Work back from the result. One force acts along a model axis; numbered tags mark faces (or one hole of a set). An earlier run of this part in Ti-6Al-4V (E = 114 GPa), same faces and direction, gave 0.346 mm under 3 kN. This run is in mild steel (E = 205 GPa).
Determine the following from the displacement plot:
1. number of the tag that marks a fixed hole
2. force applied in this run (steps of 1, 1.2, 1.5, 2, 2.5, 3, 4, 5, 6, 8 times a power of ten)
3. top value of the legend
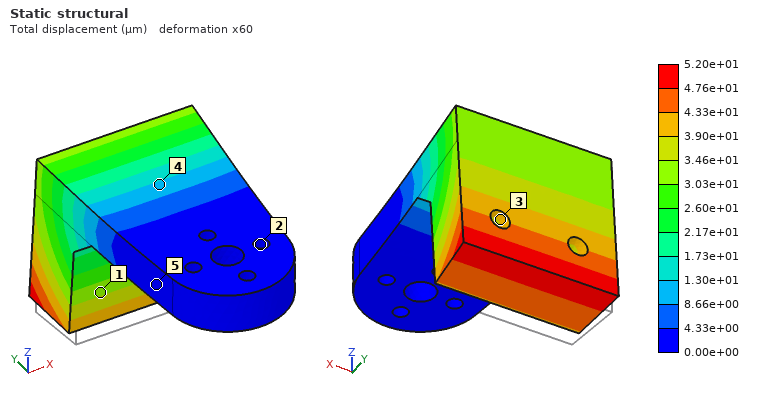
2
800 N
5.20e+01 µm
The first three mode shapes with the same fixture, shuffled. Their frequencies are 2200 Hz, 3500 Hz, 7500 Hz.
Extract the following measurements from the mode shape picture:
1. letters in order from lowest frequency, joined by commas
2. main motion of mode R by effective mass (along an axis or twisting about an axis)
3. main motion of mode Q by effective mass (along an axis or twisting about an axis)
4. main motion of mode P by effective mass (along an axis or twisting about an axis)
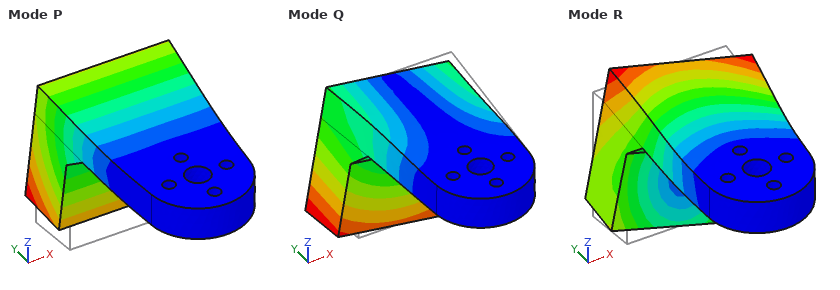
P, Q, R
along X
along X
along Z
